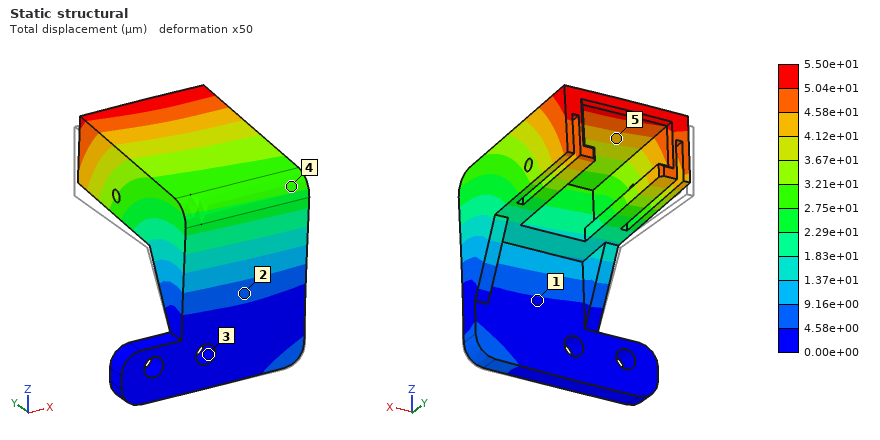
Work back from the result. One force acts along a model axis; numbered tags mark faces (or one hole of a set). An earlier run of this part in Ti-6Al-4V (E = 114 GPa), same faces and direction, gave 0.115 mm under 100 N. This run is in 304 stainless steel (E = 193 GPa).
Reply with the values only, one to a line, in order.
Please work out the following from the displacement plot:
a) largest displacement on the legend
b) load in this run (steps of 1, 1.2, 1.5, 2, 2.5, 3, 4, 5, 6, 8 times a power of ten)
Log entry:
5.50e+01 µm
80 N
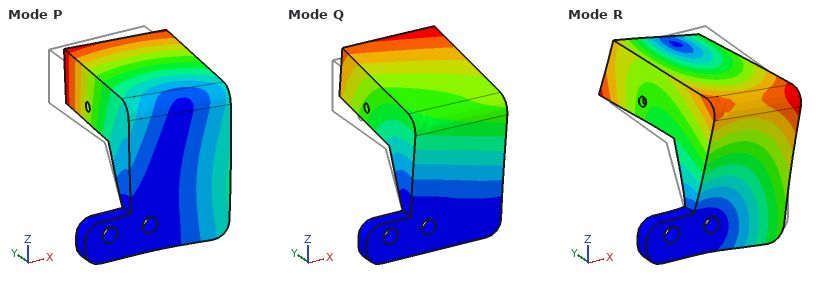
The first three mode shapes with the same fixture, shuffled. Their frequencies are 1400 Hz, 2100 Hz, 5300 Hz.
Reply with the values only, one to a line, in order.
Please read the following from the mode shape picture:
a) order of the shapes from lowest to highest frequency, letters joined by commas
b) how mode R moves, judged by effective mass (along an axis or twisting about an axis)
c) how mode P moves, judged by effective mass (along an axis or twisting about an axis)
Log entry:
Q, P, R
along X
along X
